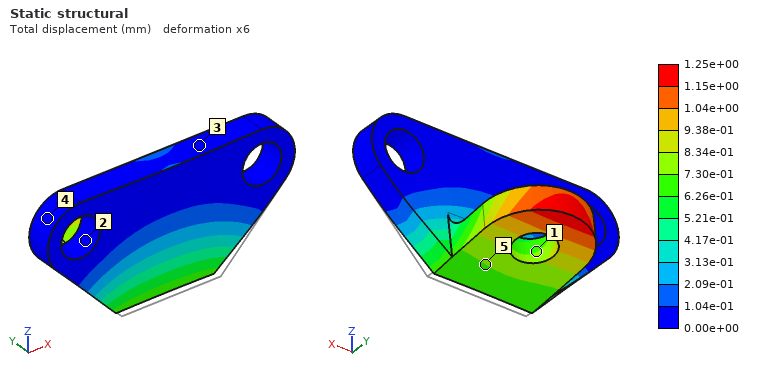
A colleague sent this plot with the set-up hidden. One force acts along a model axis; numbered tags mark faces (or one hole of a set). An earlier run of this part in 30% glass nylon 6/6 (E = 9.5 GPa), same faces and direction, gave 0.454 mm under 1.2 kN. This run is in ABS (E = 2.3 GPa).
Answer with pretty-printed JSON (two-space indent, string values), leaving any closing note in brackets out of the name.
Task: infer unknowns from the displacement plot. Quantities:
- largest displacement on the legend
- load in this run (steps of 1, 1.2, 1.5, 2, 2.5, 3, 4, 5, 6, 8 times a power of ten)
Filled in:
{
  "largest displacement on the legend": "1.25e+00 mm",
  "load in this run": "800 N"
}
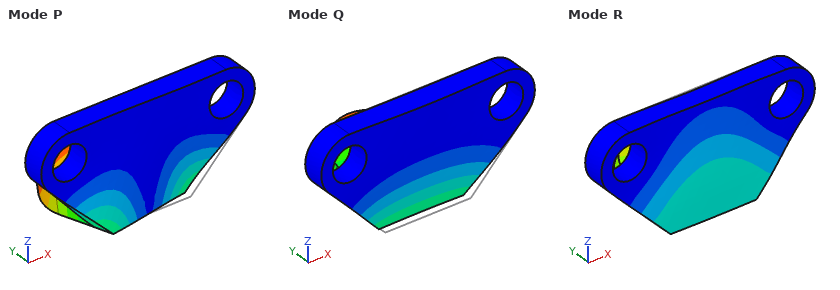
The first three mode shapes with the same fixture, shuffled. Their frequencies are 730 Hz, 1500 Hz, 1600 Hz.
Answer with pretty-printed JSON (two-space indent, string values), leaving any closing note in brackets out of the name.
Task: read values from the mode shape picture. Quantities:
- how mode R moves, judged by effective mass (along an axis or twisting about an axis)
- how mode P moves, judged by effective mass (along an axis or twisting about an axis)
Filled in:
{
  "how mode R moves, judged by effective mass": "along Y",
  "how mode P moves, judged by effective mass": "along X"
}
